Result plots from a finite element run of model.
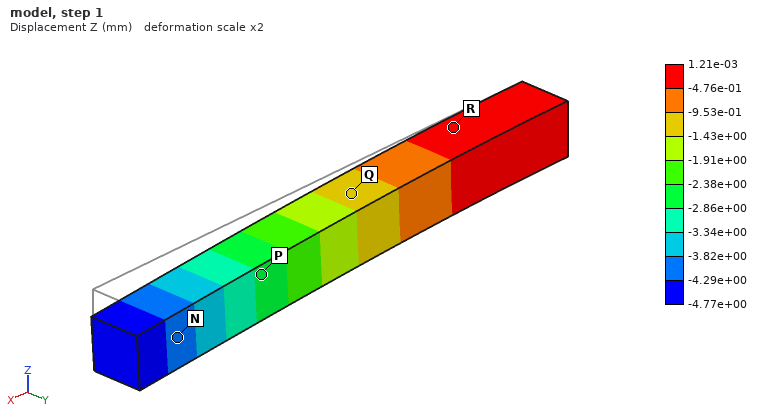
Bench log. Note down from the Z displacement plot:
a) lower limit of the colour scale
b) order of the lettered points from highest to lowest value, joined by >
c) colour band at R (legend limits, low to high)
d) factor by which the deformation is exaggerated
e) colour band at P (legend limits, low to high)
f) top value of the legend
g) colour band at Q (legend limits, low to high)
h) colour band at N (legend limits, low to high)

-4.77e+00 mm
R > Q > P > N
-4.76e-01 to 1.21e-03 mm
2
-2.86e+00 to -2.38e+00 mm
1.21e-03 mm
-1.43e+00 to -9.53e-01 mm
-4.29e+00 to -3.82e+00 mm
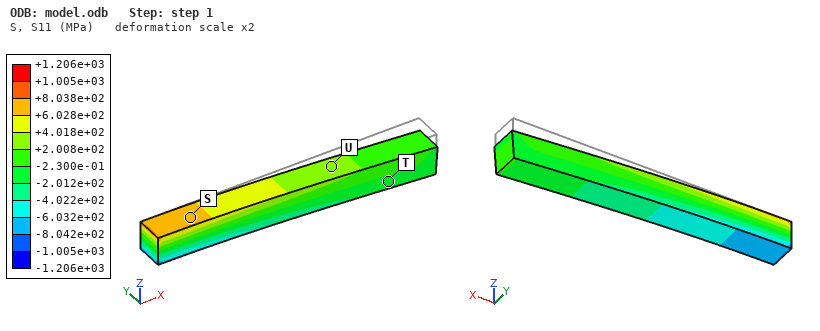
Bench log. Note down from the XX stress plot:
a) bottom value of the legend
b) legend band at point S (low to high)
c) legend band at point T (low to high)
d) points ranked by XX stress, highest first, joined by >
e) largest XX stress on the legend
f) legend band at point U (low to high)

-1.206e+03 MPa
+6.028e+02 to +8.038e+02 MPa
-2.012e+02 to -2.300e-01 MPa
S > U > T
+1.206e+03 MPa
+2.008e+02 to +4.018e+02 MPa
